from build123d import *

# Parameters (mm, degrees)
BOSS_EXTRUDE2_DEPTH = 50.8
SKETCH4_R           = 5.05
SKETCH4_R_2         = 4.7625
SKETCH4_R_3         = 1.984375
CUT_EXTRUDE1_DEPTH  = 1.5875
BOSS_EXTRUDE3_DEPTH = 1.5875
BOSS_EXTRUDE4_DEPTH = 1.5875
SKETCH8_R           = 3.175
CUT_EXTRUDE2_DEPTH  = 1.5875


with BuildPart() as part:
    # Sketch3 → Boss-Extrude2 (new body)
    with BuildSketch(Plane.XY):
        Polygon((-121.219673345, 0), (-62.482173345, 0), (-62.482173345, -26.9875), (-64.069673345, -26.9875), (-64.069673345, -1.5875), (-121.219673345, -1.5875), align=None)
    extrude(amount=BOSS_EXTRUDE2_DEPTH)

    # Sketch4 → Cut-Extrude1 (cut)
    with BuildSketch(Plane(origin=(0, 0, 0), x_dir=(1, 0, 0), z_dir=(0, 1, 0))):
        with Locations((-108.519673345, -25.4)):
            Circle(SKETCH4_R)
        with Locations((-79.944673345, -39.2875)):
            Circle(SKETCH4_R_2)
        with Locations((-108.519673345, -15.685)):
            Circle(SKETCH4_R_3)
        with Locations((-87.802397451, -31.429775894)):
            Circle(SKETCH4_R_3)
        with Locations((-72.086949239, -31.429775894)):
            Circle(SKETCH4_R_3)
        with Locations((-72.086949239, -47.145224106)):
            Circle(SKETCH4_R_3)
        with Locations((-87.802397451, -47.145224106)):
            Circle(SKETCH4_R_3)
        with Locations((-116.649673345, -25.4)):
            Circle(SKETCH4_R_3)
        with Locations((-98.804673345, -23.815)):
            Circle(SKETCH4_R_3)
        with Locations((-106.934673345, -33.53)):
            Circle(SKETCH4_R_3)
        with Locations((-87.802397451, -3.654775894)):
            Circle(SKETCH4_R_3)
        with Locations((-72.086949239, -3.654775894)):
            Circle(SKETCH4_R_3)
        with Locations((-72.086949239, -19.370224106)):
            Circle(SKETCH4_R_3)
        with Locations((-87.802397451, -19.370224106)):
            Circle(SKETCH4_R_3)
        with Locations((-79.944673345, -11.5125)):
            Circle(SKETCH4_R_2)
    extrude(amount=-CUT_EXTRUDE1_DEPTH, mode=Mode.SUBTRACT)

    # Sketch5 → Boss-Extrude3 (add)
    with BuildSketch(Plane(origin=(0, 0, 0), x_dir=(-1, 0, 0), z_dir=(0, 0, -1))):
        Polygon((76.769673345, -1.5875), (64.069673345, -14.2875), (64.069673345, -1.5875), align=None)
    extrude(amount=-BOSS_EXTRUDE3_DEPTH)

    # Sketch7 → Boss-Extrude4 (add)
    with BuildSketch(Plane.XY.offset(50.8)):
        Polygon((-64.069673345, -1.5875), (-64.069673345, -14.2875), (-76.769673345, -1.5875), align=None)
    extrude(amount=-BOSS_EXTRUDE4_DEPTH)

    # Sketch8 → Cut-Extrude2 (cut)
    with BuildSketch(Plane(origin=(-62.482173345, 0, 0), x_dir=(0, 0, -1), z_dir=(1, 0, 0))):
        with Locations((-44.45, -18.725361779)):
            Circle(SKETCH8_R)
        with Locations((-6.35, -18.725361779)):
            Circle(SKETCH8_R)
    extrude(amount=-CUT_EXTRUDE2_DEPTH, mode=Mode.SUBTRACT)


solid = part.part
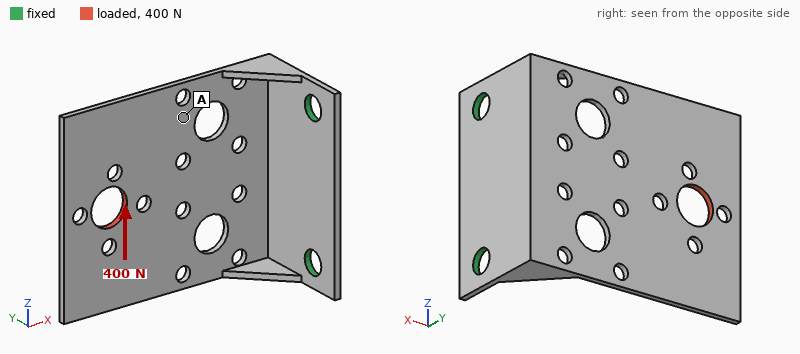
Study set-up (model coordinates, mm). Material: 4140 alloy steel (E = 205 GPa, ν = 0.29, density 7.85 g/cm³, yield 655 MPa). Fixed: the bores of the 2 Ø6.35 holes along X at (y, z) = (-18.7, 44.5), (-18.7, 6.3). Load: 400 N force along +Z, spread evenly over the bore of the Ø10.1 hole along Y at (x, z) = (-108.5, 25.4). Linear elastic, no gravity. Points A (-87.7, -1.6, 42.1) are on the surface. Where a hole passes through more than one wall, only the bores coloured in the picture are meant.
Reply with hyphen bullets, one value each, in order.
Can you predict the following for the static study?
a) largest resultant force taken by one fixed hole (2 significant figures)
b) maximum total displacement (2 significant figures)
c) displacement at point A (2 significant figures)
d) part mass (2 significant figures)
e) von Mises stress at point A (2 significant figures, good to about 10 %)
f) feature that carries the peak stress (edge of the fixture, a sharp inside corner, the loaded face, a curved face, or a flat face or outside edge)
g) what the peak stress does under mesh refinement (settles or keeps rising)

- 500 N
- 0.76 mm
- 0.38 mm
- 50 g
- 81 MPa
- edge of the fixture
- keeps rising
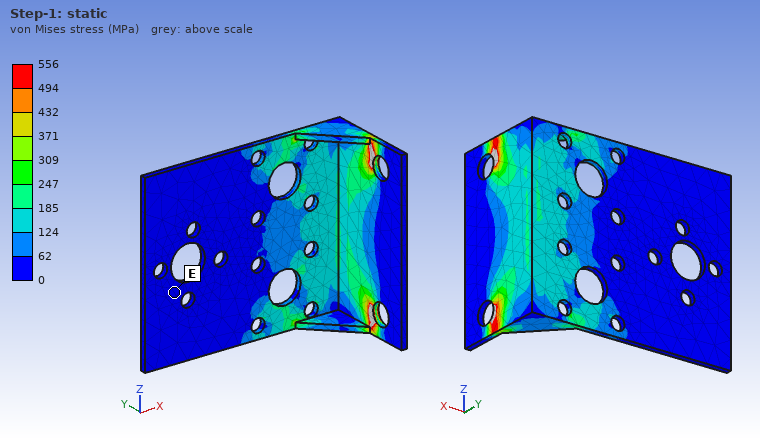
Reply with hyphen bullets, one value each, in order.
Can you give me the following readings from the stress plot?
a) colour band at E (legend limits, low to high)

- 0 to 62 MPa
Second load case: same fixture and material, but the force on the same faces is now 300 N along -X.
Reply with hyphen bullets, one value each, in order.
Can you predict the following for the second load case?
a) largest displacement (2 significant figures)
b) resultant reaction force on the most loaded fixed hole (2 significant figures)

- 0.51 mm
- 150 N
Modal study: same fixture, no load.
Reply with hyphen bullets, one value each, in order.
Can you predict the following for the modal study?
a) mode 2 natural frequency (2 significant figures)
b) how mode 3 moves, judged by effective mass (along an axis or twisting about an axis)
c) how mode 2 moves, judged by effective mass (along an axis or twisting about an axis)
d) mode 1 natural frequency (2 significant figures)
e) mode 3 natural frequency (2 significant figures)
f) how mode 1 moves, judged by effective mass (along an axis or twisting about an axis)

- 830 Hz
- along Z
- along Z
- 340 Hz
- 1400 Hz
- along Y
